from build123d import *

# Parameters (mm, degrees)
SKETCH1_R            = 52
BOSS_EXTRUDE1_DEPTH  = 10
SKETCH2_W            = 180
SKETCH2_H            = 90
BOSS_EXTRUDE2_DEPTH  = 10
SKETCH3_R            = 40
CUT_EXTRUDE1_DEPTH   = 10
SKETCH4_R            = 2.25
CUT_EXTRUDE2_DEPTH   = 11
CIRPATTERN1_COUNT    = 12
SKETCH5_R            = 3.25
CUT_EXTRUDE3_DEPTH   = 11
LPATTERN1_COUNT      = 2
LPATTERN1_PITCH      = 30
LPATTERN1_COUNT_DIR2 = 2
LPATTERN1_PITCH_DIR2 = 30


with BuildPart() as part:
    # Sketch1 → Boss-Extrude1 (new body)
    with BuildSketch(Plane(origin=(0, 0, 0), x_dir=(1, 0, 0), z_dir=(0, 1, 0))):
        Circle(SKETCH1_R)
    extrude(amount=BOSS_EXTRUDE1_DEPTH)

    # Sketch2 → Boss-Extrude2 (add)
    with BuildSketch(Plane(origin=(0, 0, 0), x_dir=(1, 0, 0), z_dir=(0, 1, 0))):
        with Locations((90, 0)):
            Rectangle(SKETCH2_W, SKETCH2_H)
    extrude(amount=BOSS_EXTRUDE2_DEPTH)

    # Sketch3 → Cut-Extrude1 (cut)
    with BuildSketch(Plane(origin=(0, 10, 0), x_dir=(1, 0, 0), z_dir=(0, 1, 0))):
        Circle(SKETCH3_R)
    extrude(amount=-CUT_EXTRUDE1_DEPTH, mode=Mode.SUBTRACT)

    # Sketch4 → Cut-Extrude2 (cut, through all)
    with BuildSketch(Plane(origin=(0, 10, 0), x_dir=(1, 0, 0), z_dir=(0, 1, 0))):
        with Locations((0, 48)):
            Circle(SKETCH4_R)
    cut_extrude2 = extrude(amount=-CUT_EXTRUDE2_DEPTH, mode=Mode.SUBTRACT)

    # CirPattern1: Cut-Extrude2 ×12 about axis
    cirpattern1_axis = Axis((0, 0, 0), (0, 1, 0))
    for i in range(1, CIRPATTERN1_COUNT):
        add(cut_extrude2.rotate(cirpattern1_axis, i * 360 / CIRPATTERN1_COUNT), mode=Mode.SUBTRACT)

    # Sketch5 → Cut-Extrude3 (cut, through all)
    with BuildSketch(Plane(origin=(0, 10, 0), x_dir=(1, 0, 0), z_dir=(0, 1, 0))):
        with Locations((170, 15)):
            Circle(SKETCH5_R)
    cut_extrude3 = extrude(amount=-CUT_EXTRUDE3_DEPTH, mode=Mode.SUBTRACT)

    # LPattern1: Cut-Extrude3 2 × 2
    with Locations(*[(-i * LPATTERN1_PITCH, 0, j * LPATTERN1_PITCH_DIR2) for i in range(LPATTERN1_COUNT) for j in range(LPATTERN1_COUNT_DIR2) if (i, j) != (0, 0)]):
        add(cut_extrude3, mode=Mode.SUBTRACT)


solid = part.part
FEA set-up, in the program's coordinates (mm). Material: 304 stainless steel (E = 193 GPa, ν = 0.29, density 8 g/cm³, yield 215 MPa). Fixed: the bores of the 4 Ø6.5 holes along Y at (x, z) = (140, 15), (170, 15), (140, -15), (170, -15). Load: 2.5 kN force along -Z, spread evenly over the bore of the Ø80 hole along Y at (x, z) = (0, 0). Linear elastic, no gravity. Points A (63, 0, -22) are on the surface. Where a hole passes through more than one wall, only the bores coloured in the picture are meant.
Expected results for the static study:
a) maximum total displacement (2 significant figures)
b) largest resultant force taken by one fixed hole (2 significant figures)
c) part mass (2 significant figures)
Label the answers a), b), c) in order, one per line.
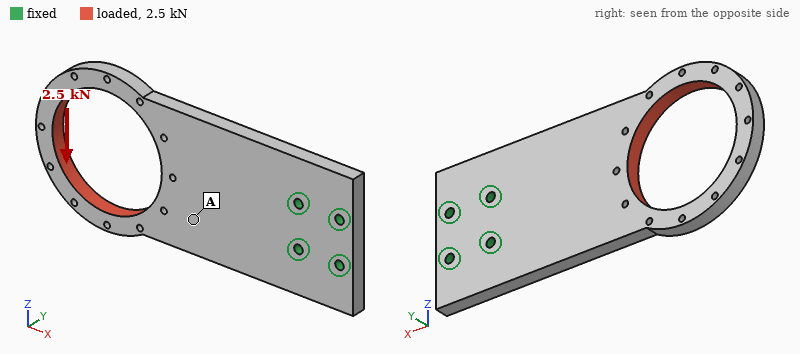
a) 0.14 mm
b) 5.9 kN
c) 1.2 kg
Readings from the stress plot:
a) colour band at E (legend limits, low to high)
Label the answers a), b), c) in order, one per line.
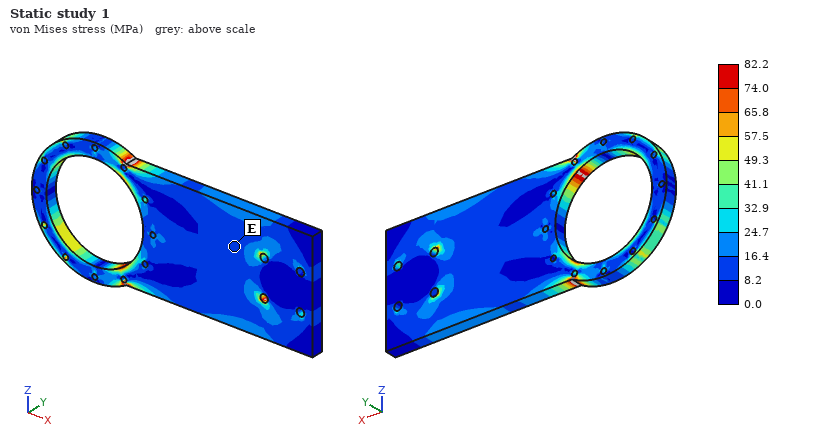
a) 8.2 to 16.4 MPa
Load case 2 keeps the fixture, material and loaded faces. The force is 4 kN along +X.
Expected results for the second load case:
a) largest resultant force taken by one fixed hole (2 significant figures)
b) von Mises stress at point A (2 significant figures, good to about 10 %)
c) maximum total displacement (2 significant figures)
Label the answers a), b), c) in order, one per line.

a) 1.6 kN
b) 4.5 MPa
c) 26 µm
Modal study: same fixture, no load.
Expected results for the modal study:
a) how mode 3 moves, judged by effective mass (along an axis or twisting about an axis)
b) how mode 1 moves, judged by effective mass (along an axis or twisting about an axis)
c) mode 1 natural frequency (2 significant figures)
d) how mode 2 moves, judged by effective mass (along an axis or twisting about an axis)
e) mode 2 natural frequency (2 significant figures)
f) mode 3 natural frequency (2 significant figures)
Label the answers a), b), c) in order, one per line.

a) along Y
b) along Y
c) 320 Hz
d) twisting about X
e) 940 Hz
f) 1100 Hz
